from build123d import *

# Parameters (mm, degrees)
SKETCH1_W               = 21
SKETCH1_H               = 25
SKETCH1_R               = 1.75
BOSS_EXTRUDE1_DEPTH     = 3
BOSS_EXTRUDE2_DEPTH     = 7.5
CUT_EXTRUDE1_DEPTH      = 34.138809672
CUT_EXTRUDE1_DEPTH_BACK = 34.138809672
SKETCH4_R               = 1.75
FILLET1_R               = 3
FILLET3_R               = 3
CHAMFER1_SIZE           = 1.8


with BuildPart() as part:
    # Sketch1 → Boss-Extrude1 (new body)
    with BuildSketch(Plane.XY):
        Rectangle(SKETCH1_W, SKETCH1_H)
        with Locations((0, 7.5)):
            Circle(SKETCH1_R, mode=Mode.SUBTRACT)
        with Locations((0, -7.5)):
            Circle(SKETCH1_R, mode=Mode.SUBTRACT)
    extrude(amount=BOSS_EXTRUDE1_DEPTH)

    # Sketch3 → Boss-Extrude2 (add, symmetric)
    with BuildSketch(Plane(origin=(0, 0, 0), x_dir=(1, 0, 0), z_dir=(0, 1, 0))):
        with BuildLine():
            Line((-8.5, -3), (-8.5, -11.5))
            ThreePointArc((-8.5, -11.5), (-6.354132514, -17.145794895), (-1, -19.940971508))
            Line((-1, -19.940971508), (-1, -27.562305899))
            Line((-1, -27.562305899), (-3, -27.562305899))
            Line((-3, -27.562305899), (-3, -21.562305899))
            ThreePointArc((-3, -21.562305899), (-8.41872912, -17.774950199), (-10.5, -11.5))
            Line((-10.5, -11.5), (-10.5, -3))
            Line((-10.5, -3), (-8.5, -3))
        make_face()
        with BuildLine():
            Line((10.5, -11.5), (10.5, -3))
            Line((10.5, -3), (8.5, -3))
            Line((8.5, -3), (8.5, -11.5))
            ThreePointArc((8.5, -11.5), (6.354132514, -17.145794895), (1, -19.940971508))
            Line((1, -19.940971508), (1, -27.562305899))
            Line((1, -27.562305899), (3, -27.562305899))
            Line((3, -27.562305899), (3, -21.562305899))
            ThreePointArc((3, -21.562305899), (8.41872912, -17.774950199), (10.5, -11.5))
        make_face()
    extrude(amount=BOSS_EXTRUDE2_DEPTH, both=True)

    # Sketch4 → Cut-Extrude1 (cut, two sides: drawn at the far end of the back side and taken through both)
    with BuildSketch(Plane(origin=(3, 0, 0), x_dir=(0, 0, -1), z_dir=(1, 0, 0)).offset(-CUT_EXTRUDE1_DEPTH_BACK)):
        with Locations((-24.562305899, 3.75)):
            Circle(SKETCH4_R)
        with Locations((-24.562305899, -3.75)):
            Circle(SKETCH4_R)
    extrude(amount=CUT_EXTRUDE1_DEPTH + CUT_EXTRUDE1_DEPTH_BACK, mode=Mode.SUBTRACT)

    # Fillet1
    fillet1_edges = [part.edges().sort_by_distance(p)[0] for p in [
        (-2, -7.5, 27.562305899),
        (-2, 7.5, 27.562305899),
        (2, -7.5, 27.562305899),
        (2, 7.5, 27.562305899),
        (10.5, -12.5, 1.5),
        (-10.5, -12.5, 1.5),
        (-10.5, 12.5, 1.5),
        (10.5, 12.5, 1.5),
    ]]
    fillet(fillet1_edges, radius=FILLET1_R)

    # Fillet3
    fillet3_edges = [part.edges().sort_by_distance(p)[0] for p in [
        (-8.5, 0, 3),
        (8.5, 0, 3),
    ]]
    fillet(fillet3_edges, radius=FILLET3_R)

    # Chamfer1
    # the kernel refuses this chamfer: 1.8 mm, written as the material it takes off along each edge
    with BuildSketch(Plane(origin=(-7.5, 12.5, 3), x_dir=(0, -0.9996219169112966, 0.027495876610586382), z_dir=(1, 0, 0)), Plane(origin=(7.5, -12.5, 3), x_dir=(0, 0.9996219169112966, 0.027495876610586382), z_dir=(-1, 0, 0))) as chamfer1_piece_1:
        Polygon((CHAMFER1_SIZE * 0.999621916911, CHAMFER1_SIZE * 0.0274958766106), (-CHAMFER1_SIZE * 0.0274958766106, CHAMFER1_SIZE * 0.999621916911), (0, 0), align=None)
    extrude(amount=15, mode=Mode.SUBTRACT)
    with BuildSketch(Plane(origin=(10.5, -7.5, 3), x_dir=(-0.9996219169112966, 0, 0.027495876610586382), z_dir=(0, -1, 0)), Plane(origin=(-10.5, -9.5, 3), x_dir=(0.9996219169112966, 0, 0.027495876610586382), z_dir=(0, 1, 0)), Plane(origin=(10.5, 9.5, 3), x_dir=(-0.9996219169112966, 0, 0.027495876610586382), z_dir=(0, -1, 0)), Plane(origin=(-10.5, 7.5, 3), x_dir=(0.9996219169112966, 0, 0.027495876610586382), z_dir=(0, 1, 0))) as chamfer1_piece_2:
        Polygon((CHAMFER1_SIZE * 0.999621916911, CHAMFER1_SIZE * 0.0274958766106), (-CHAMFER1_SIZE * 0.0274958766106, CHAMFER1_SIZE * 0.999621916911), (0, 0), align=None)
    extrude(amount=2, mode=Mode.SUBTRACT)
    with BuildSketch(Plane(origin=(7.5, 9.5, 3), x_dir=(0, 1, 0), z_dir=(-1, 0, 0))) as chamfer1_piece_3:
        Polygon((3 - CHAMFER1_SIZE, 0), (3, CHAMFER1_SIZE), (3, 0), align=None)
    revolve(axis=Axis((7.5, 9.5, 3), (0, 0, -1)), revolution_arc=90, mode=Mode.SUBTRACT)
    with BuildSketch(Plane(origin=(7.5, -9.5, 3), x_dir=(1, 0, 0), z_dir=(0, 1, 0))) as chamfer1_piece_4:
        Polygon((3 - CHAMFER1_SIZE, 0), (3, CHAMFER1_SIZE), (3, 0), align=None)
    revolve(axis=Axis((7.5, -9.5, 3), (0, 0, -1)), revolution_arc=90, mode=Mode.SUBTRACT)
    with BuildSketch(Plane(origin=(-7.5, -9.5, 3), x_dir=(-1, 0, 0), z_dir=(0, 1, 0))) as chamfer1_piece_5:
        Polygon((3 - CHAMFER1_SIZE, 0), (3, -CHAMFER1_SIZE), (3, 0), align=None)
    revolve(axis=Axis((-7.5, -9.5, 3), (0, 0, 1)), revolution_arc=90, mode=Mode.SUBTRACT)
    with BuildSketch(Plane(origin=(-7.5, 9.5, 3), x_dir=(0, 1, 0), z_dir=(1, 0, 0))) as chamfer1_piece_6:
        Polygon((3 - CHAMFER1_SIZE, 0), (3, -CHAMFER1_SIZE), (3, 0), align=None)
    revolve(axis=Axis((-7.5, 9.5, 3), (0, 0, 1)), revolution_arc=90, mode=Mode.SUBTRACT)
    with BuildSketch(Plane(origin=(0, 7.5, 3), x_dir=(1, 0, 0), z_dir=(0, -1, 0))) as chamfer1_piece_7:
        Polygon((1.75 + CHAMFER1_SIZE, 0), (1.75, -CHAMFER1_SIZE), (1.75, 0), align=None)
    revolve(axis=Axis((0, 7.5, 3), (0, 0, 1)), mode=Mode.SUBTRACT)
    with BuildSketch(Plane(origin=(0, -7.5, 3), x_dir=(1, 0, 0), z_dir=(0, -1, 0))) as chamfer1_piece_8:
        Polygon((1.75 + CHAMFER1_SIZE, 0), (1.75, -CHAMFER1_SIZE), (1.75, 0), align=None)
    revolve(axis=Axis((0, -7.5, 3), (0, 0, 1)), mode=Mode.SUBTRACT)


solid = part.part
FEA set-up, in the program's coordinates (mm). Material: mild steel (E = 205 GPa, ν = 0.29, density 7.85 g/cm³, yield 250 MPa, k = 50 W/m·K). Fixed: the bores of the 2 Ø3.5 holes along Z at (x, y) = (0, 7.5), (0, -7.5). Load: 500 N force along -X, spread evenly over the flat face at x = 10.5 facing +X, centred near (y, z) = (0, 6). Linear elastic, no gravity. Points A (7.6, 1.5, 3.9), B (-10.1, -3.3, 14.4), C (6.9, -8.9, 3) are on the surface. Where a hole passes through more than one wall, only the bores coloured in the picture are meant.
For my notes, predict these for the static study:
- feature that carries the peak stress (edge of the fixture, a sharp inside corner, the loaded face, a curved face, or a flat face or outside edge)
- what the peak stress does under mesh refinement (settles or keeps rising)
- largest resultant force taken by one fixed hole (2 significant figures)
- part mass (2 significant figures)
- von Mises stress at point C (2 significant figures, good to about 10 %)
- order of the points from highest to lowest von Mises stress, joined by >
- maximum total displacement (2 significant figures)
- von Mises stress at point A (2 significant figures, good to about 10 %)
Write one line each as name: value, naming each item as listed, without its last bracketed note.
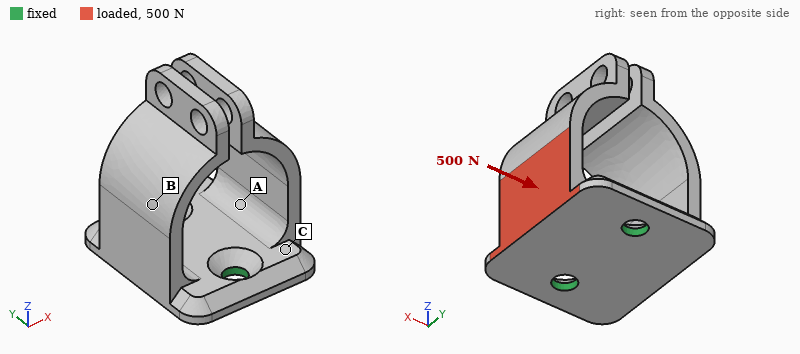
feature that carries the peak stress: edge of the fixture
what the peak stress does under mesh refinement: keeps rising
largest resultant force taken by one fixed hole: 250 N
part mass: 24 g
von Mises stress at point C: 37 MPa
order of the points from highest to lowest von Mises stress, joined by >: A > C > B
maximum total displacement: 0.10 mm
von Mises stress at point A: 82 MPa
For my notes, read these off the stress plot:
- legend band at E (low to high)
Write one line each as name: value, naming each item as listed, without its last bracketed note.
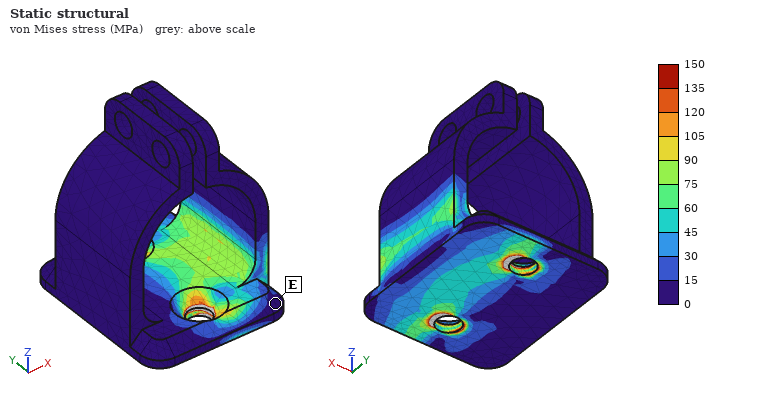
legend band at E: 0 to 15 MPa
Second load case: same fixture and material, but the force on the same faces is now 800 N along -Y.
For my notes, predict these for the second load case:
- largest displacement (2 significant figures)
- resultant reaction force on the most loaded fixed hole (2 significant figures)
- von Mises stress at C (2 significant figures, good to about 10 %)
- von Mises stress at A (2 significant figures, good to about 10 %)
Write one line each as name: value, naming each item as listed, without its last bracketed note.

largest displacement: 24 µm
resultant reaction force on the most loaded fixed hole: 690 N
von Mises stress at C: 32 MPa
von Mises stress at A: 74 MPa
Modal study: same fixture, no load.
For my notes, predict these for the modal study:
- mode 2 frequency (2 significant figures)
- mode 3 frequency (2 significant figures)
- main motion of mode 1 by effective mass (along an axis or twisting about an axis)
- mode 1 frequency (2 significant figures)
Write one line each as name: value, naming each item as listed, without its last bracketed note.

mode 2 frequency: 2300 Hz
mode 3 frequency: 4700 Hz
main motion of mode 1 by effective mass: along X
mode 1 frequency: 2200 Hz
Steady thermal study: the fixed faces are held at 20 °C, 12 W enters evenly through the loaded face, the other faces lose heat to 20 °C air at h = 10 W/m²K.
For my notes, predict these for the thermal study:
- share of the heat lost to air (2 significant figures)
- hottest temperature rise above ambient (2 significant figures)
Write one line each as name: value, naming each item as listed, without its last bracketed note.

share of the heat lost to air: 5.4 %
hottest temperature rise above ambient: 59 K
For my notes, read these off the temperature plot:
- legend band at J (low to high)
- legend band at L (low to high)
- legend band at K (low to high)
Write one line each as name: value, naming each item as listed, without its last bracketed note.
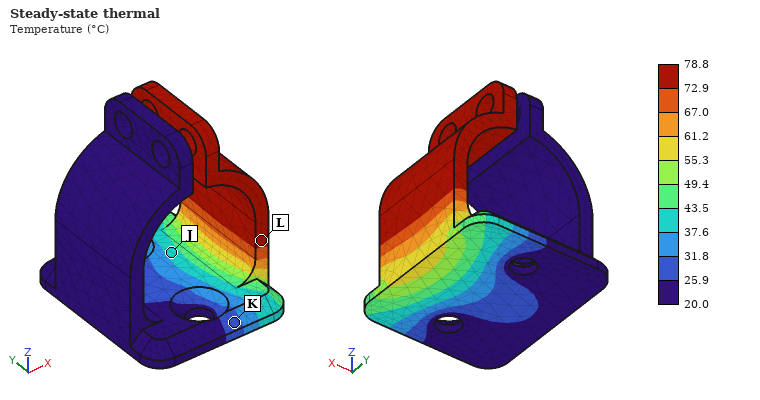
legend band at J: 37.6 to 43.5 °C
legend band at L: 72.9 to 78.8 °C
legend band at K: 25.9 to 31.8 °C
